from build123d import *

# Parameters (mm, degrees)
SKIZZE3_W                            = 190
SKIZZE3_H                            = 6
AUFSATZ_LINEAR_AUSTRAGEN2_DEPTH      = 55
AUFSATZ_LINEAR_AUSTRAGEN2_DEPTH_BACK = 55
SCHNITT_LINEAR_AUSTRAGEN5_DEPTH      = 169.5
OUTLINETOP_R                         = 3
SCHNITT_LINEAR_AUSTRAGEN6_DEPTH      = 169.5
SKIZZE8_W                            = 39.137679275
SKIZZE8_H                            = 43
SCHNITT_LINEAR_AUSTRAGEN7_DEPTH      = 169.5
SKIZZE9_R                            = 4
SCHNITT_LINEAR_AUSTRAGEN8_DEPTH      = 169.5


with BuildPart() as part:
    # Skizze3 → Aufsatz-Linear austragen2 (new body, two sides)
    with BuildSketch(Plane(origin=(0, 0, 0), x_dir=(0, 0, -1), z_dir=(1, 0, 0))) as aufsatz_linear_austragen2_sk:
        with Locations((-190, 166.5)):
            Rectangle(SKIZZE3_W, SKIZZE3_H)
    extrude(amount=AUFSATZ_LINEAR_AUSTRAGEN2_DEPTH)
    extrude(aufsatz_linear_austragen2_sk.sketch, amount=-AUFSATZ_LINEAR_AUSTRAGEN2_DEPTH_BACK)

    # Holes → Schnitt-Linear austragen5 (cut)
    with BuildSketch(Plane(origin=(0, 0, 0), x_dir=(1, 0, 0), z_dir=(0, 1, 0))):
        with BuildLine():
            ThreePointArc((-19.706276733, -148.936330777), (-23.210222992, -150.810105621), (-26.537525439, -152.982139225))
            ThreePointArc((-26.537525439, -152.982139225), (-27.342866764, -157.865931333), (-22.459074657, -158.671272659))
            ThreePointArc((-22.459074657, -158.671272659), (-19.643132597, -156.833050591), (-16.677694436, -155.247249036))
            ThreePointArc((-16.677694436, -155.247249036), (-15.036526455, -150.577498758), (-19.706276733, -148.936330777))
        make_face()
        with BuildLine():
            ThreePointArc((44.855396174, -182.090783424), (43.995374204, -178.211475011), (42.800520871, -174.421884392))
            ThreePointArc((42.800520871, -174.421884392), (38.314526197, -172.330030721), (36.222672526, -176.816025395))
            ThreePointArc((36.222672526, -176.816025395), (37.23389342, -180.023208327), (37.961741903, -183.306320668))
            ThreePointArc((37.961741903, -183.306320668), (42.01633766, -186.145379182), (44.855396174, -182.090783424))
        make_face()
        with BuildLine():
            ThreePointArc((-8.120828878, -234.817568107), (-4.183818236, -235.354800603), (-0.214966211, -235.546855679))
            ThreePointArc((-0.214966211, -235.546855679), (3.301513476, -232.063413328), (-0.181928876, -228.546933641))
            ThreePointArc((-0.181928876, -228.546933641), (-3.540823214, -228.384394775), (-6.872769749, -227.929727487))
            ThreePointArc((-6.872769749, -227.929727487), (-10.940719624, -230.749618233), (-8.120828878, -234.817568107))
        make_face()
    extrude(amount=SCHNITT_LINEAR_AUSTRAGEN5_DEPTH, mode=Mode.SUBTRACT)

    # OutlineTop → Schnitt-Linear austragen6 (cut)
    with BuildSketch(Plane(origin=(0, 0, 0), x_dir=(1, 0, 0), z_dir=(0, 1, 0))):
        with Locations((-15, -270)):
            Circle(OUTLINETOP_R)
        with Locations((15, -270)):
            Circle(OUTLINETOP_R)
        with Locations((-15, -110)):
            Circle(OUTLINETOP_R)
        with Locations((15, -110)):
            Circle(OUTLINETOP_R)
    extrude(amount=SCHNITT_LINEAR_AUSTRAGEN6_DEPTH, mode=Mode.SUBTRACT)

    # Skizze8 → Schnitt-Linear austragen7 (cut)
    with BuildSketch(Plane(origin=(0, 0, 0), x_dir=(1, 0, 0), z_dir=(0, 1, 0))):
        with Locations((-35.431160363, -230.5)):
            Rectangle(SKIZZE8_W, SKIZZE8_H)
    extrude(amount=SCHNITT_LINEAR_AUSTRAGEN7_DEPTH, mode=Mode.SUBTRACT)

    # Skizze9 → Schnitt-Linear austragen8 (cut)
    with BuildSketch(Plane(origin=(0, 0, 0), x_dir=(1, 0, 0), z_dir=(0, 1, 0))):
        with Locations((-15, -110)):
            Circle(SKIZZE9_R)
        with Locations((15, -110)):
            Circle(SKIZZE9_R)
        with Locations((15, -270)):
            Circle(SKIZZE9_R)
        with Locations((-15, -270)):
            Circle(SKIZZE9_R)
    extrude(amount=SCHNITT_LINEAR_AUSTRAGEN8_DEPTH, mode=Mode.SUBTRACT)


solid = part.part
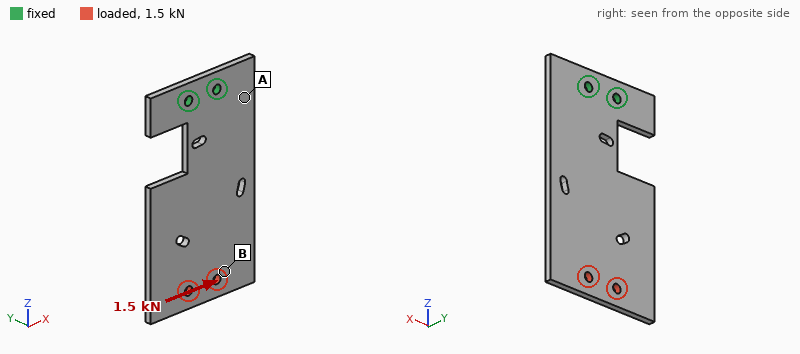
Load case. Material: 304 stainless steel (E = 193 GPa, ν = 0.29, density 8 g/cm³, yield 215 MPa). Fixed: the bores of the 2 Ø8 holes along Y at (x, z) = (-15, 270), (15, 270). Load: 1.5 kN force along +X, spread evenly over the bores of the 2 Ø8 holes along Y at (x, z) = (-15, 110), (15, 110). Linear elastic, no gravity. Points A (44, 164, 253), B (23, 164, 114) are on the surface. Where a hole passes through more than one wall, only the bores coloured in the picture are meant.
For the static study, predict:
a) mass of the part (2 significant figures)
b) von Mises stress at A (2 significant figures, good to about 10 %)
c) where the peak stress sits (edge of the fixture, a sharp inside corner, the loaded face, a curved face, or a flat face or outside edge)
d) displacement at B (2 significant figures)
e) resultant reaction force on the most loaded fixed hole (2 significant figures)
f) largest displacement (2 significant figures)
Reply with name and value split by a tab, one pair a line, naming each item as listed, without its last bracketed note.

mass of the part	900 g
von Mises stress at A	22 MPa
where the peak stress sits	edge of the fixture
displacement at B	0.12 mm
resultant reaction force on the most loaded fixed hole	6.9 kN
largest displacement	0.15 mm
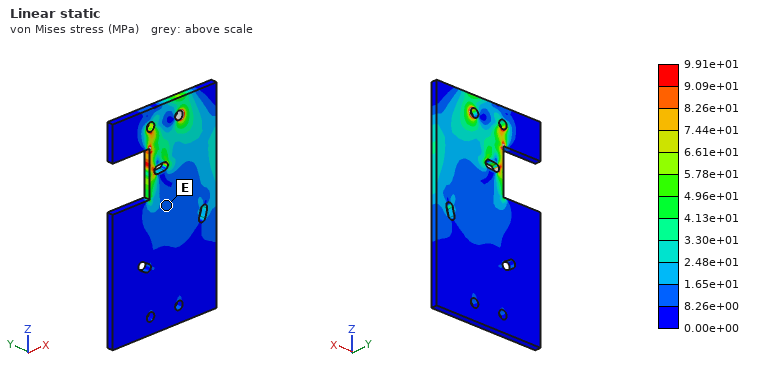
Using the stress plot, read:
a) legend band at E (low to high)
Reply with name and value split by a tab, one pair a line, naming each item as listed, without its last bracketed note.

legend band at E	8.26e+00 to 1.65e+01 MPa
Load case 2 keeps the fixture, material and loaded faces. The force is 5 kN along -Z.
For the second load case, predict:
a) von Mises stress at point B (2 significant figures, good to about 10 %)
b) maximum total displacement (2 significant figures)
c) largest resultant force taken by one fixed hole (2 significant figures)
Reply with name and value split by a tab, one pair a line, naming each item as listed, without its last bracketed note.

von Mises stress at point B	13 MPa
maximum total displacement	47 µm
largest resultant force taken by one fixed hole	2.6 kN
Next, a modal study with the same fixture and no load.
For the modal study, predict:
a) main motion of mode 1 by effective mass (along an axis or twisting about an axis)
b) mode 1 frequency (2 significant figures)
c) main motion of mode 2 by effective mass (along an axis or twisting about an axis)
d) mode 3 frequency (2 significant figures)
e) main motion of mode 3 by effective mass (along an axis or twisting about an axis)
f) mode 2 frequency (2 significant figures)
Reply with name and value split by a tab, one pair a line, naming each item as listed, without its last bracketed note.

main motion of mode 1 by effective mass	along Y
mode 1 frequency	120 Hz
main motion of mode 2 by effective mass	twisting about Z
mode 3 frequency	860 Hz
main motion of mode 3 by effective mass	along Y
mode 2 frequency	400 Hz
